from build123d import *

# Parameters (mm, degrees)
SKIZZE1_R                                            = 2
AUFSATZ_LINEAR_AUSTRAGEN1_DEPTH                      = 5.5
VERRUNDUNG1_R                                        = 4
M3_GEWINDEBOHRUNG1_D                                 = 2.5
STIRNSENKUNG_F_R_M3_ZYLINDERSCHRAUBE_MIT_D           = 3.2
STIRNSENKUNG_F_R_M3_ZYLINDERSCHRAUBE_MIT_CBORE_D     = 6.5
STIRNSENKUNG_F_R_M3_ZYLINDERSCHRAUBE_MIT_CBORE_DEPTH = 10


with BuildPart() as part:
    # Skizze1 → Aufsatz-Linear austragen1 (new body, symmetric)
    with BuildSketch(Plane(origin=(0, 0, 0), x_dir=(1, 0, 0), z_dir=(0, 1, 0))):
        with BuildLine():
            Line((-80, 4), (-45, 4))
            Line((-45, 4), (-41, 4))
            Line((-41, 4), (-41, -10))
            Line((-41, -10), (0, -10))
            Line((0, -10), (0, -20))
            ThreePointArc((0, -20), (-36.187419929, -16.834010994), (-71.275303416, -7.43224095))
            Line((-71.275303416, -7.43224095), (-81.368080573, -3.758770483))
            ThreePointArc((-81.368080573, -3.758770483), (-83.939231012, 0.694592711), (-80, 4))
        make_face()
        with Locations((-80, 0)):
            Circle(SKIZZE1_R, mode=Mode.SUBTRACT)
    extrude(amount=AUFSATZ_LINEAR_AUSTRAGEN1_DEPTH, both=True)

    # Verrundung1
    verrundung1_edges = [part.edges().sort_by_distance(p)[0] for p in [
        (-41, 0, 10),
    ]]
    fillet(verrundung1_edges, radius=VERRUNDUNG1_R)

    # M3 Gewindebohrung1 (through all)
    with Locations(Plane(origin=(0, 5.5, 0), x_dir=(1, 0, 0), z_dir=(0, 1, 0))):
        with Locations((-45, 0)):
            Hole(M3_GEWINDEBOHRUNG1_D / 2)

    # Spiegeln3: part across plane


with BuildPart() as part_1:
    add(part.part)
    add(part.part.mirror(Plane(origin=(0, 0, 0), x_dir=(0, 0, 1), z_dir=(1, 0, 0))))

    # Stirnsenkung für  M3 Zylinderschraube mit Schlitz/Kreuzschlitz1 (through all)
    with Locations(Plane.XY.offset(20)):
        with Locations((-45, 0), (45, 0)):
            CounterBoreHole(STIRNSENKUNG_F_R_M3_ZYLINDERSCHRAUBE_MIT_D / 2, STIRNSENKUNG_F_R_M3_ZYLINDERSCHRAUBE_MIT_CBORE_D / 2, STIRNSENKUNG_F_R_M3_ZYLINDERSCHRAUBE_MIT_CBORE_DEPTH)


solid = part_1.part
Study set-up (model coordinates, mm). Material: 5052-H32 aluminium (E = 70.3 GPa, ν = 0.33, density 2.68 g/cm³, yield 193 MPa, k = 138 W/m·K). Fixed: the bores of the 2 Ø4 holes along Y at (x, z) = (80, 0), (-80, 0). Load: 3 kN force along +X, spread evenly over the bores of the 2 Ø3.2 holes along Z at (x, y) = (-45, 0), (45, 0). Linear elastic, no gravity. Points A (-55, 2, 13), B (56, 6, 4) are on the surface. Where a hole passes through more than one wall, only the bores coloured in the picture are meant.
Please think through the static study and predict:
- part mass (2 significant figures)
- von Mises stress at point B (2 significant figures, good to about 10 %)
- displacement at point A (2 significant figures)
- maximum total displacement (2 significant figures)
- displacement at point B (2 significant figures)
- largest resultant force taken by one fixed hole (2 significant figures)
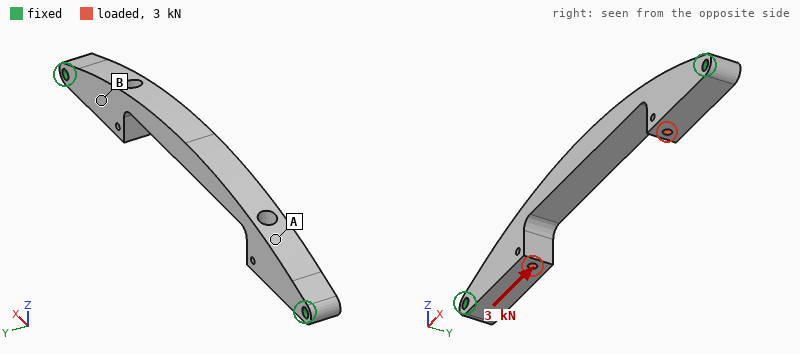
54 g
10.0 MPa
16 µm
20 µm
13 µm
1.5 kN
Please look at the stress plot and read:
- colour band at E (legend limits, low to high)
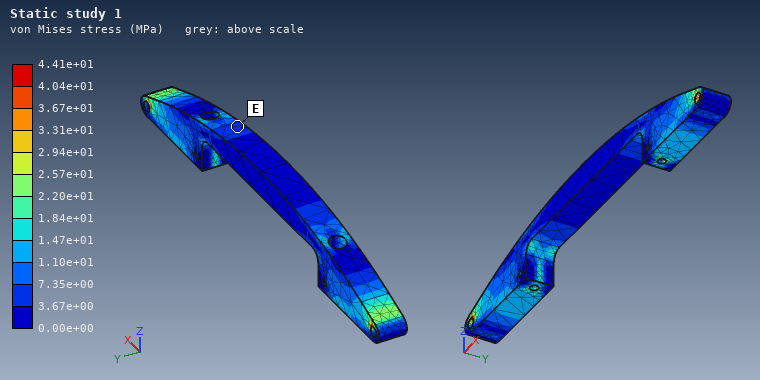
3.67e+00 to 7.35e+00 MPa
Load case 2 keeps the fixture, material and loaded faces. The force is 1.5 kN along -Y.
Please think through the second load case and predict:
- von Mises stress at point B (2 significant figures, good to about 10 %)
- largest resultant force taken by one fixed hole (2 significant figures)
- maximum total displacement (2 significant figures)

13 MPa
750 N
0.17 mm
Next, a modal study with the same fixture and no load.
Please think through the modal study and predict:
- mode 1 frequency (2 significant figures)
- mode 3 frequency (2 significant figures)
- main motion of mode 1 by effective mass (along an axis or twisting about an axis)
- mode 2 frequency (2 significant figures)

2100 Hz
3700 Hz
along Y
3700 Hz
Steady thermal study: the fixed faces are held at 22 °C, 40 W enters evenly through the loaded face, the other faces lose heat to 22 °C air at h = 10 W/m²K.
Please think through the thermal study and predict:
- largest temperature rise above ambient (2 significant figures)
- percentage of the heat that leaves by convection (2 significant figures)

36 K
5.1 %
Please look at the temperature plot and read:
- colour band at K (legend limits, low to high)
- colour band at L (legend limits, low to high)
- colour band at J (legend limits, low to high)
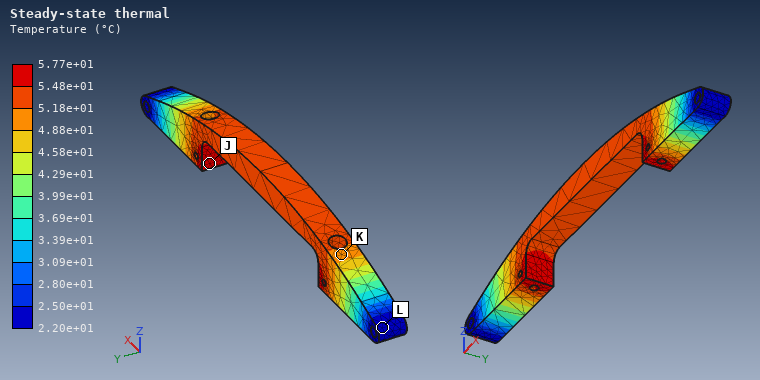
4.88e+01 to 5.18e+01 °C
2.20e+01 to 2.50e+01 °C
5.48e+01 to 5.77e+01 °C
